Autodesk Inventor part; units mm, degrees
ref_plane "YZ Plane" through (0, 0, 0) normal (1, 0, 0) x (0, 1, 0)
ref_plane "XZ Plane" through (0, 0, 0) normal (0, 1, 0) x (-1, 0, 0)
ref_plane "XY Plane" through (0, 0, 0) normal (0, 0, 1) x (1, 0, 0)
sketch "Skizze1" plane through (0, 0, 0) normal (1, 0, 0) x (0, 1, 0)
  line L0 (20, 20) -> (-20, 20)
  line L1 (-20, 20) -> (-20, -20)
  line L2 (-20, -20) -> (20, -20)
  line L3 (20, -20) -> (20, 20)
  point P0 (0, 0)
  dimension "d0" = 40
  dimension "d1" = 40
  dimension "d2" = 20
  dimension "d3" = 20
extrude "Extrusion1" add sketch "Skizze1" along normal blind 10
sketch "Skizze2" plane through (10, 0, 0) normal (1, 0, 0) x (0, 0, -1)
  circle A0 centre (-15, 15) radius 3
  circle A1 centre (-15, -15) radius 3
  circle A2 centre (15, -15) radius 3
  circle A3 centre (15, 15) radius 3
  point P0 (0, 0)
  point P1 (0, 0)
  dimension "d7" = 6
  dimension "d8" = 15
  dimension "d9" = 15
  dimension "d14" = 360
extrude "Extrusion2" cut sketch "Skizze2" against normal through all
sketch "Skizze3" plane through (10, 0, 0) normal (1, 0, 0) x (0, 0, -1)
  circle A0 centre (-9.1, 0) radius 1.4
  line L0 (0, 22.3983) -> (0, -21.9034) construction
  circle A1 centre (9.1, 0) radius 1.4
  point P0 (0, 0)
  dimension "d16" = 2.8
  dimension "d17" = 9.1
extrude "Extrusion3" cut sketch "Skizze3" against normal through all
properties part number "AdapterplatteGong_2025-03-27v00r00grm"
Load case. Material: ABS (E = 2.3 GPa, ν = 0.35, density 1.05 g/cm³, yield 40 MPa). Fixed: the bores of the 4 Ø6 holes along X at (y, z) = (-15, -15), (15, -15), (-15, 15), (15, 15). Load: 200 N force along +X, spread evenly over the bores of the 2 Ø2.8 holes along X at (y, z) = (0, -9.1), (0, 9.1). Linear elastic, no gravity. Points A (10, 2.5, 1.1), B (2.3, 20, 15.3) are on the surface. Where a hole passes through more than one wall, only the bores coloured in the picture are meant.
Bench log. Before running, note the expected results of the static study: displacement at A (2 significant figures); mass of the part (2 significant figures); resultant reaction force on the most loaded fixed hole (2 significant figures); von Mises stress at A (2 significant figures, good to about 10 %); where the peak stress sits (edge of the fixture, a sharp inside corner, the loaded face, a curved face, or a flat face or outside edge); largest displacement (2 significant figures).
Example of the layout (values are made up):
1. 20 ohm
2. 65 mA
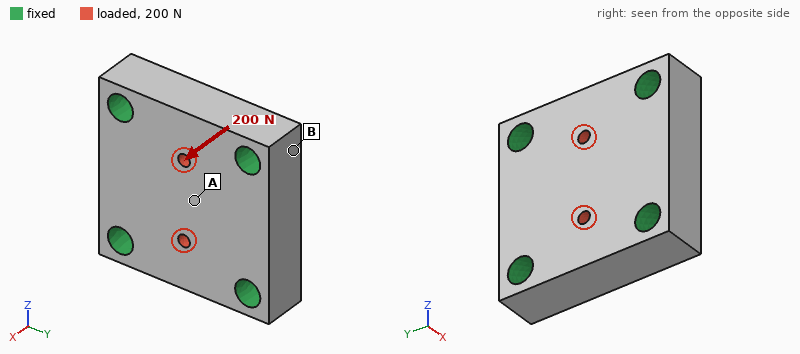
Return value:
1. 9.7 µm
2. 15 g
3. 50 N
4. 0.87 MPa
5. the loaded face
6. 13 µm
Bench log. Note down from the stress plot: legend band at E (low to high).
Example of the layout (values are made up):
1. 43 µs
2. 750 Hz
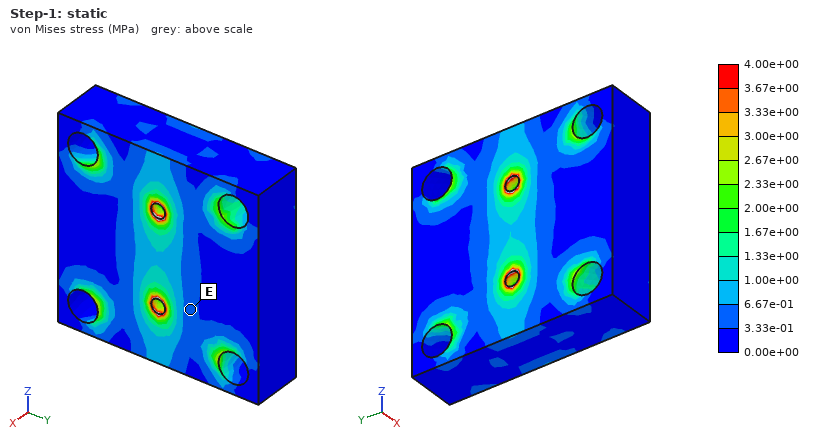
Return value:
1. 3.33e-01 to 6.67e-01 MPa
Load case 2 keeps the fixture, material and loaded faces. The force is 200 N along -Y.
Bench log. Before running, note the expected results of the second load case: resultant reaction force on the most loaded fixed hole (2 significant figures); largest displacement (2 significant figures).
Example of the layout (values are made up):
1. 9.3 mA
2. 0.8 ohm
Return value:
1. 53 N
2. 3.9 µm
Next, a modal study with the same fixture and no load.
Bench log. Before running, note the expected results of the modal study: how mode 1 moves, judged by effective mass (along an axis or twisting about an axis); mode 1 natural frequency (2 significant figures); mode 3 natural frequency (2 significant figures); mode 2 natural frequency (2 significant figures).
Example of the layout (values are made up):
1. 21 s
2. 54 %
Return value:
1. along X
2. 9400 Hz
3. 13 kHz
4. 13 kHz
